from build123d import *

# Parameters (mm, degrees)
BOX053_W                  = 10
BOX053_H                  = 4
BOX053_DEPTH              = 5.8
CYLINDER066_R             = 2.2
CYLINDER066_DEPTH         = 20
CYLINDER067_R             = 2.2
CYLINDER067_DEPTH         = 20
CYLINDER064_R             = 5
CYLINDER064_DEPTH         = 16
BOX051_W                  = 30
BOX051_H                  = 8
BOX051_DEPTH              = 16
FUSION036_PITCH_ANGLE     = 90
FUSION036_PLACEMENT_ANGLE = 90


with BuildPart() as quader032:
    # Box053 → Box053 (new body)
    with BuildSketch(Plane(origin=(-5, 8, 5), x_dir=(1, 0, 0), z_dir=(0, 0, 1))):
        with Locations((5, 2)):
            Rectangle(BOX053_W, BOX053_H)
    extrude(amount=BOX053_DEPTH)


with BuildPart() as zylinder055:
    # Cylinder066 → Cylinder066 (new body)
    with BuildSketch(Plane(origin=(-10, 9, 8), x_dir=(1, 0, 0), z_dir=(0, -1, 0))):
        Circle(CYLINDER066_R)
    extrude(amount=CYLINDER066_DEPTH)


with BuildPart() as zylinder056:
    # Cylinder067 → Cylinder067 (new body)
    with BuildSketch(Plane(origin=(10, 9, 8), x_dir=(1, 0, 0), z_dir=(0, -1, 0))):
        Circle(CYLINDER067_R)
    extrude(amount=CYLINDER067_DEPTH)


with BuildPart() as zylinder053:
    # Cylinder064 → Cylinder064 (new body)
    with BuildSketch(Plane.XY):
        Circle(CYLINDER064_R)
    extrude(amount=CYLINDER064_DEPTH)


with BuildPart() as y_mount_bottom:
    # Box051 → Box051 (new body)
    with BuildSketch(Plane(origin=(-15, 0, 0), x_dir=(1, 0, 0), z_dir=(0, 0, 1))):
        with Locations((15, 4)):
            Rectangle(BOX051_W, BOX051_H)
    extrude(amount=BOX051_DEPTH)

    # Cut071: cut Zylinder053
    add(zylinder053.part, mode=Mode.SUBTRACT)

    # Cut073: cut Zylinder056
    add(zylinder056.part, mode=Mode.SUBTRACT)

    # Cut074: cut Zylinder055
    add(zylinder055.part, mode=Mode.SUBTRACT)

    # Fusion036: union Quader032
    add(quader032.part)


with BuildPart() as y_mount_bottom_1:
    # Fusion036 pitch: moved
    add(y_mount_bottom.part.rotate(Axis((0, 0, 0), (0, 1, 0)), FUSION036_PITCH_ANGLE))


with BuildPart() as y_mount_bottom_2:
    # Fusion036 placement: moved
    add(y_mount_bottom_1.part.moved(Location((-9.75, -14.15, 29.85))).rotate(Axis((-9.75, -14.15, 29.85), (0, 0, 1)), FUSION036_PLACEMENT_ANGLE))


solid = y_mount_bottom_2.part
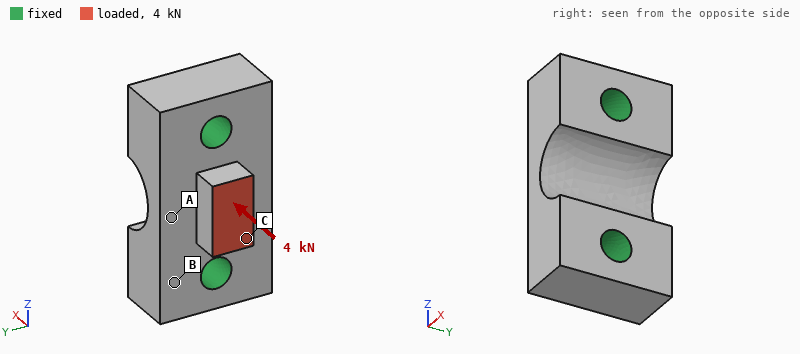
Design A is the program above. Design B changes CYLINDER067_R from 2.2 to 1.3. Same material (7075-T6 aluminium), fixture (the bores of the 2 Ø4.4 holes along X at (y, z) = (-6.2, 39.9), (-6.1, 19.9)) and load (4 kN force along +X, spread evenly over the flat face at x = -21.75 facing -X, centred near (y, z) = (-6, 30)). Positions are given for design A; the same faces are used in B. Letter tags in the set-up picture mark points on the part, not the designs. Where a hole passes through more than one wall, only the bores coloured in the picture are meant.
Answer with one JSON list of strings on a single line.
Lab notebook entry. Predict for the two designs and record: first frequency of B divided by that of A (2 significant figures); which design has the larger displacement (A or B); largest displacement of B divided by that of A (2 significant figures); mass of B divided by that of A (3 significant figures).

["0.89", "B", "1.1", "1.02"]
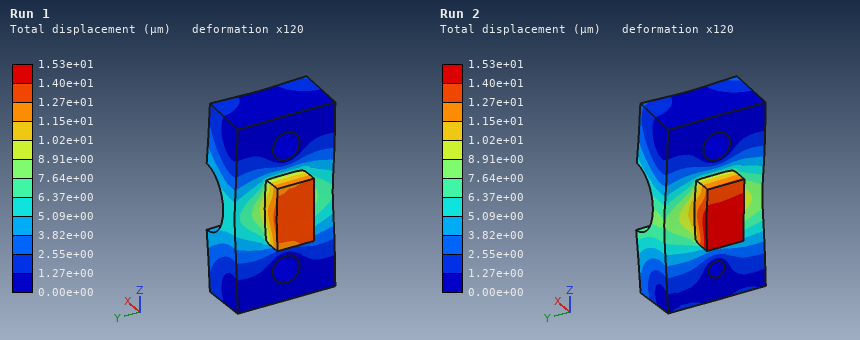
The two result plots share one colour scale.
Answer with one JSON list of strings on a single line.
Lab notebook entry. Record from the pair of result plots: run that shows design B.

["Run 2"]
